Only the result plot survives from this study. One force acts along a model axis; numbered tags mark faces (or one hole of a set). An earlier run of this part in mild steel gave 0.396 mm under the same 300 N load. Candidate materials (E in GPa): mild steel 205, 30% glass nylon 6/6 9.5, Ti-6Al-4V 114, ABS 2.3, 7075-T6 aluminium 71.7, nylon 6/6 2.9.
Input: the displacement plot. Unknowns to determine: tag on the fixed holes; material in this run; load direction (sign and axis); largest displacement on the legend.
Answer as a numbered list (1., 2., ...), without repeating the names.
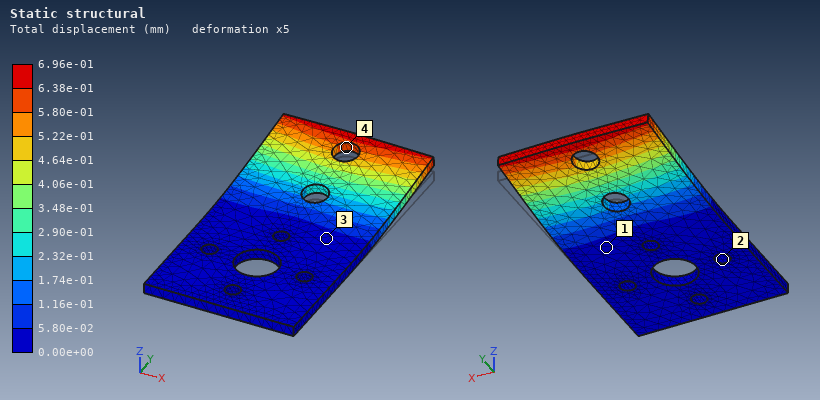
1. 2
2. Ti-6Al-4V
3. +Z
4. 6.96e-01 mm
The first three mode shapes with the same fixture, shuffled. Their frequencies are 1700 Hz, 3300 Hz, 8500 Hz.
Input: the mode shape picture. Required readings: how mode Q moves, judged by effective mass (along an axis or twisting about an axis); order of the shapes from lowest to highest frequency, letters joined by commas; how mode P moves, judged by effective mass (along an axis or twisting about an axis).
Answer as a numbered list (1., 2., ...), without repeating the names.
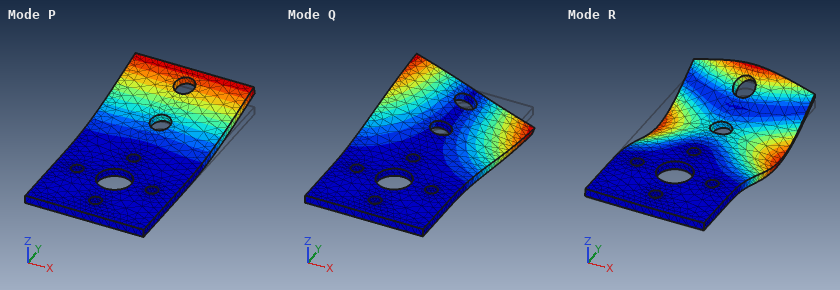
1. twisting about Y
2. P, Q, R
3. along Z
